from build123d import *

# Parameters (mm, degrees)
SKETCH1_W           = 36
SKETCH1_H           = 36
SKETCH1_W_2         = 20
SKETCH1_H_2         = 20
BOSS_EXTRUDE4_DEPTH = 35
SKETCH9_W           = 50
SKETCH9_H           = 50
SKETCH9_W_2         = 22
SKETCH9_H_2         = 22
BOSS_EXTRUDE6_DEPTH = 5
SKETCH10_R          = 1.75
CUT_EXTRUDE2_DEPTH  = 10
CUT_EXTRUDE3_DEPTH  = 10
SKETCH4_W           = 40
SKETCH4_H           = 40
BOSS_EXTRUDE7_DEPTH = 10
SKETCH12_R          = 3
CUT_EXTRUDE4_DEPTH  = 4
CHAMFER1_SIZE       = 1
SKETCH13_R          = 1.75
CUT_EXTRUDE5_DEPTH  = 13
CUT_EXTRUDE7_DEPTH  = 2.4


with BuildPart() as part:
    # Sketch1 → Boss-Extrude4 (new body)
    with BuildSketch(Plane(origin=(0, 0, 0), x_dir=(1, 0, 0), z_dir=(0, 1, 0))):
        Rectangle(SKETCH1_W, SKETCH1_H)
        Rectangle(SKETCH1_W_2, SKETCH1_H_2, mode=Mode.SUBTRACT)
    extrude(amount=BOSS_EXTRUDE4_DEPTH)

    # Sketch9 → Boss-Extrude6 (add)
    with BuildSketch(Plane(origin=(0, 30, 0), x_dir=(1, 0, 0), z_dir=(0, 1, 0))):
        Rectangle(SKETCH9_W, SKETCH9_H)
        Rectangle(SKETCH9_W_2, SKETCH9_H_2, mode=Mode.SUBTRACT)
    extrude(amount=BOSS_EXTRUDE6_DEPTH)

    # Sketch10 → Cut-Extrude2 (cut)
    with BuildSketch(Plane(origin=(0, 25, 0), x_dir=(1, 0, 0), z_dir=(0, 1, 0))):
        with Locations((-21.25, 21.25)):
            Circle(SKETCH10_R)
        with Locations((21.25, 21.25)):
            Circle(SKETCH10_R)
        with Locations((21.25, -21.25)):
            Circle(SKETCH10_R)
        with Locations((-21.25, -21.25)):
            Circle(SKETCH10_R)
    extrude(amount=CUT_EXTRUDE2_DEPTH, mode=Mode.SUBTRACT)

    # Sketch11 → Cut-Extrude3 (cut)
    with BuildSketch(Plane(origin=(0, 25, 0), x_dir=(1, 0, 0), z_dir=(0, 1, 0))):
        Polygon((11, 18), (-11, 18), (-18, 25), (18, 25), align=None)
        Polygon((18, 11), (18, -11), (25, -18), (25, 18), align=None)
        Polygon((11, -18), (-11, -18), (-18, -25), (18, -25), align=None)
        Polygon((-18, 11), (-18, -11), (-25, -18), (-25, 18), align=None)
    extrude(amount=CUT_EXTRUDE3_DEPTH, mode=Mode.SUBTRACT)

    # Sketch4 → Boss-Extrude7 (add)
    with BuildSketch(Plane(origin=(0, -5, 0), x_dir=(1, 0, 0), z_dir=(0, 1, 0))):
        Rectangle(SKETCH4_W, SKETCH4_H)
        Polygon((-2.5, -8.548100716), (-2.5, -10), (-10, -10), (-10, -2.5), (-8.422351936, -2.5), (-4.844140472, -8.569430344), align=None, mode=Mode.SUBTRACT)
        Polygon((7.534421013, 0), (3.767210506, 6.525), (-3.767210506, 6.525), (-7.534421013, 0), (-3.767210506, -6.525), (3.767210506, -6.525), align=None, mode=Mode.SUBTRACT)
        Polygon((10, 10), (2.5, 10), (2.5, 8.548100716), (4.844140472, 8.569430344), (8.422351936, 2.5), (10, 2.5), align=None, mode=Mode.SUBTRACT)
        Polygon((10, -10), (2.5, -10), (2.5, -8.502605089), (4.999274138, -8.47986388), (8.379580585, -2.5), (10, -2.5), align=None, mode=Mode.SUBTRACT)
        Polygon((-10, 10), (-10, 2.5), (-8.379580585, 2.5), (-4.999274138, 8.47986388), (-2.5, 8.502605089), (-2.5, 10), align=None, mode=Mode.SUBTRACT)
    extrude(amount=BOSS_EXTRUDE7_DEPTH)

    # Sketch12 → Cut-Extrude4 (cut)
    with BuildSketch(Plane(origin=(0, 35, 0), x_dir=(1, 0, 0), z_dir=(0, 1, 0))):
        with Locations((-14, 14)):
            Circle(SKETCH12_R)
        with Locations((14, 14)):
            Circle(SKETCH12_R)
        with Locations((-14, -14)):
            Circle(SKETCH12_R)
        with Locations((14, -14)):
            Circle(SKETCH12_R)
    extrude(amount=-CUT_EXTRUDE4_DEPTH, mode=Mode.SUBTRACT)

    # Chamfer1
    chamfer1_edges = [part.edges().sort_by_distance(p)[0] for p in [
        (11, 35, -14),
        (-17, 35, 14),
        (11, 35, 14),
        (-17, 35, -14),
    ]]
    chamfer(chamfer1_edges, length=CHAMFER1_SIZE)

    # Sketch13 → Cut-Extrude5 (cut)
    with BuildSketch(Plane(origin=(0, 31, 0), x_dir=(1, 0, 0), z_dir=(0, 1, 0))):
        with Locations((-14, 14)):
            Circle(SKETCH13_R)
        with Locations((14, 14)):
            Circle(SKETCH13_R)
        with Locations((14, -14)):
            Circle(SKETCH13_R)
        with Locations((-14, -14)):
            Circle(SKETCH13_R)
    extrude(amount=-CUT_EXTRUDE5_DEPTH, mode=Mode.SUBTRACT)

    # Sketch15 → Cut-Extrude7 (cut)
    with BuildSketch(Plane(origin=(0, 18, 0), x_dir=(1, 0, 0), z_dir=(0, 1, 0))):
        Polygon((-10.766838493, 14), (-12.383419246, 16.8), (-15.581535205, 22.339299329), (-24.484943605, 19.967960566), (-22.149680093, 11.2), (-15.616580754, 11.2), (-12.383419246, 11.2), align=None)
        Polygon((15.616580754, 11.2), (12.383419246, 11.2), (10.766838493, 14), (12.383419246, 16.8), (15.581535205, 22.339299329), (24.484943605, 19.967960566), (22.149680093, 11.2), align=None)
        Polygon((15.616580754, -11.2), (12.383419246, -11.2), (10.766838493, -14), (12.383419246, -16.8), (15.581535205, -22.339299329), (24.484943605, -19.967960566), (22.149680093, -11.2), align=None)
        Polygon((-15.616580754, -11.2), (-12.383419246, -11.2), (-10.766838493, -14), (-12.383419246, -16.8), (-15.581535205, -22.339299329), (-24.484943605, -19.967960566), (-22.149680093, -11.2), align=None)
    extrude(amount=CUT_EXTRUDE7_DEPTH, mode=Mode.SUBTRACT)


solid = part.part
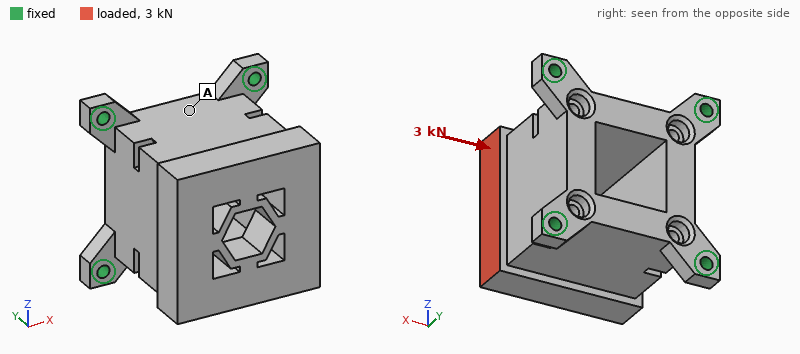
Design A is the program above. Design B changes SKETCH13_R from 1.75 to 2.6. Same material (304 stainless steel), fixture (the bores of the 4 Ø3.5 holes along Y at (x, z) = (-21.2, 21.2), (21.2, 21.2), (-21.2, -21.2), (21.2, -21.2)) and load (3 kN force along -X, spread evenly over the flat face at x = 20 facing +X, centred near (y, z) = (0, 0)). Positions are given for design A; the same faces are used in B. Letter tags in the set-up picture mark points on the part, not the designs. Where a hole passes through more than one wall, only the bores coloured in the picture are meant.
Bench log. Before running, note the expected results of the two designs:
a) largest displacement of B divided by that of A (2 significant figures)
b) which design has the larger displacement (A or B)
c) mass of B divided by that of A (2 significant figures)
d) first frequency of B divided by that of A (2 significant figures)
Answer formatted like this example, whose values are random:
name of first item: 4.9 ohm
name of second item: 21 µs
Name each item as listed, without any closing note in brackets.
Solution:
largest displacement of B divided by that of A: 1.1
which design has the larger displacement: B
mass of B divided by that of A: 0.99
first frequency of B divided by that of A: 0.95
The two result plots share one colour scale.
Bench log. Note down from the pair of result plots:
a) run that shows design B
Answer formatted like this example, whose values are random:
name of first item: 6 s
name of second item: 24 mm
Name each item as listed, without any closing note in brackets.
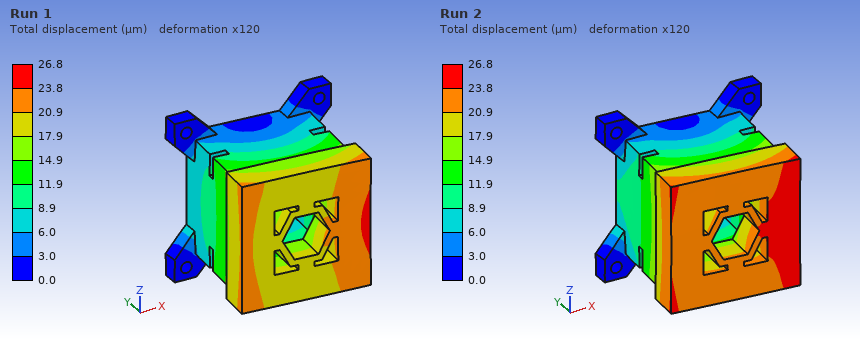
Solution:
run that shows design B: Run 2
